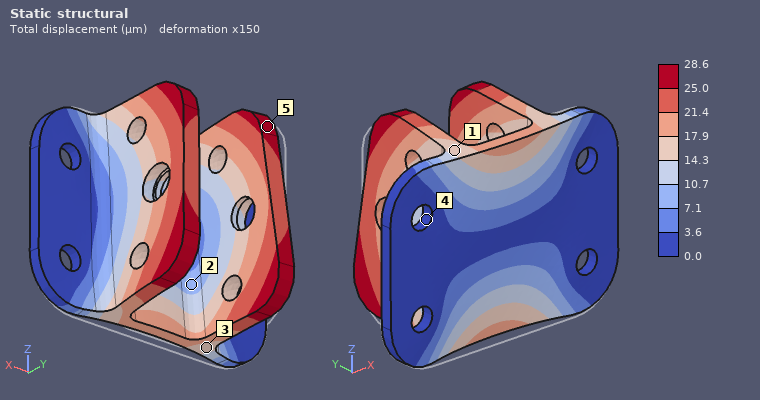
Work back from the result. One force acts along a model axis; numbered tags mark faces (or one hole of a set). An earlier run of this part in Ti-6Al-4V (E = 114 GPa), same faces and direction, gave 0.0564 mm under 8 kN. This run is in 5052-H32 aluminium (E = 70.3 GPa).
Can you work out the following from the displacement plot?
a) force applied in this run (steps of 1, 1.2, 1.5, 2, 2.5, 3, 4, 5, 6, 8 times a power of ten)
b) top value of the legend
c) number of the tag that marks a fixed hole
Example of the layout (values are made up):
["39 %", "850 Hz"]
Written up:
["2.5 kN", "28.6 µm", "4"]
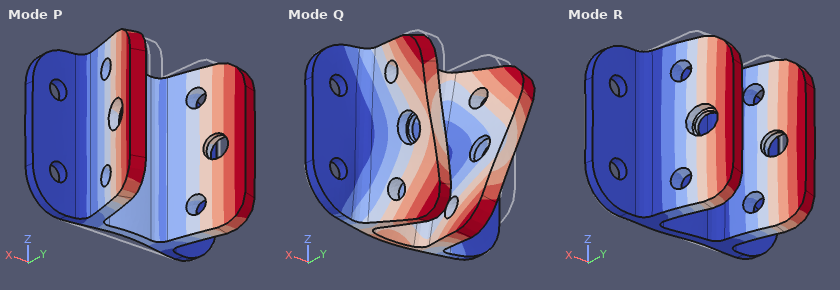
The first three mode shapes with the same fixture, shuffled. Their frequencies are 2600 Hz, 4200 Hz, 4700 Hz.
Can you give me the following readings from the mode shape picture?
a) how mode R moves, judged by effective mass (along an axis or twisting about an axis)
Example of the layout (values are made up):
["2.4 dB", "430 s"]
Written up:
["along X"]
